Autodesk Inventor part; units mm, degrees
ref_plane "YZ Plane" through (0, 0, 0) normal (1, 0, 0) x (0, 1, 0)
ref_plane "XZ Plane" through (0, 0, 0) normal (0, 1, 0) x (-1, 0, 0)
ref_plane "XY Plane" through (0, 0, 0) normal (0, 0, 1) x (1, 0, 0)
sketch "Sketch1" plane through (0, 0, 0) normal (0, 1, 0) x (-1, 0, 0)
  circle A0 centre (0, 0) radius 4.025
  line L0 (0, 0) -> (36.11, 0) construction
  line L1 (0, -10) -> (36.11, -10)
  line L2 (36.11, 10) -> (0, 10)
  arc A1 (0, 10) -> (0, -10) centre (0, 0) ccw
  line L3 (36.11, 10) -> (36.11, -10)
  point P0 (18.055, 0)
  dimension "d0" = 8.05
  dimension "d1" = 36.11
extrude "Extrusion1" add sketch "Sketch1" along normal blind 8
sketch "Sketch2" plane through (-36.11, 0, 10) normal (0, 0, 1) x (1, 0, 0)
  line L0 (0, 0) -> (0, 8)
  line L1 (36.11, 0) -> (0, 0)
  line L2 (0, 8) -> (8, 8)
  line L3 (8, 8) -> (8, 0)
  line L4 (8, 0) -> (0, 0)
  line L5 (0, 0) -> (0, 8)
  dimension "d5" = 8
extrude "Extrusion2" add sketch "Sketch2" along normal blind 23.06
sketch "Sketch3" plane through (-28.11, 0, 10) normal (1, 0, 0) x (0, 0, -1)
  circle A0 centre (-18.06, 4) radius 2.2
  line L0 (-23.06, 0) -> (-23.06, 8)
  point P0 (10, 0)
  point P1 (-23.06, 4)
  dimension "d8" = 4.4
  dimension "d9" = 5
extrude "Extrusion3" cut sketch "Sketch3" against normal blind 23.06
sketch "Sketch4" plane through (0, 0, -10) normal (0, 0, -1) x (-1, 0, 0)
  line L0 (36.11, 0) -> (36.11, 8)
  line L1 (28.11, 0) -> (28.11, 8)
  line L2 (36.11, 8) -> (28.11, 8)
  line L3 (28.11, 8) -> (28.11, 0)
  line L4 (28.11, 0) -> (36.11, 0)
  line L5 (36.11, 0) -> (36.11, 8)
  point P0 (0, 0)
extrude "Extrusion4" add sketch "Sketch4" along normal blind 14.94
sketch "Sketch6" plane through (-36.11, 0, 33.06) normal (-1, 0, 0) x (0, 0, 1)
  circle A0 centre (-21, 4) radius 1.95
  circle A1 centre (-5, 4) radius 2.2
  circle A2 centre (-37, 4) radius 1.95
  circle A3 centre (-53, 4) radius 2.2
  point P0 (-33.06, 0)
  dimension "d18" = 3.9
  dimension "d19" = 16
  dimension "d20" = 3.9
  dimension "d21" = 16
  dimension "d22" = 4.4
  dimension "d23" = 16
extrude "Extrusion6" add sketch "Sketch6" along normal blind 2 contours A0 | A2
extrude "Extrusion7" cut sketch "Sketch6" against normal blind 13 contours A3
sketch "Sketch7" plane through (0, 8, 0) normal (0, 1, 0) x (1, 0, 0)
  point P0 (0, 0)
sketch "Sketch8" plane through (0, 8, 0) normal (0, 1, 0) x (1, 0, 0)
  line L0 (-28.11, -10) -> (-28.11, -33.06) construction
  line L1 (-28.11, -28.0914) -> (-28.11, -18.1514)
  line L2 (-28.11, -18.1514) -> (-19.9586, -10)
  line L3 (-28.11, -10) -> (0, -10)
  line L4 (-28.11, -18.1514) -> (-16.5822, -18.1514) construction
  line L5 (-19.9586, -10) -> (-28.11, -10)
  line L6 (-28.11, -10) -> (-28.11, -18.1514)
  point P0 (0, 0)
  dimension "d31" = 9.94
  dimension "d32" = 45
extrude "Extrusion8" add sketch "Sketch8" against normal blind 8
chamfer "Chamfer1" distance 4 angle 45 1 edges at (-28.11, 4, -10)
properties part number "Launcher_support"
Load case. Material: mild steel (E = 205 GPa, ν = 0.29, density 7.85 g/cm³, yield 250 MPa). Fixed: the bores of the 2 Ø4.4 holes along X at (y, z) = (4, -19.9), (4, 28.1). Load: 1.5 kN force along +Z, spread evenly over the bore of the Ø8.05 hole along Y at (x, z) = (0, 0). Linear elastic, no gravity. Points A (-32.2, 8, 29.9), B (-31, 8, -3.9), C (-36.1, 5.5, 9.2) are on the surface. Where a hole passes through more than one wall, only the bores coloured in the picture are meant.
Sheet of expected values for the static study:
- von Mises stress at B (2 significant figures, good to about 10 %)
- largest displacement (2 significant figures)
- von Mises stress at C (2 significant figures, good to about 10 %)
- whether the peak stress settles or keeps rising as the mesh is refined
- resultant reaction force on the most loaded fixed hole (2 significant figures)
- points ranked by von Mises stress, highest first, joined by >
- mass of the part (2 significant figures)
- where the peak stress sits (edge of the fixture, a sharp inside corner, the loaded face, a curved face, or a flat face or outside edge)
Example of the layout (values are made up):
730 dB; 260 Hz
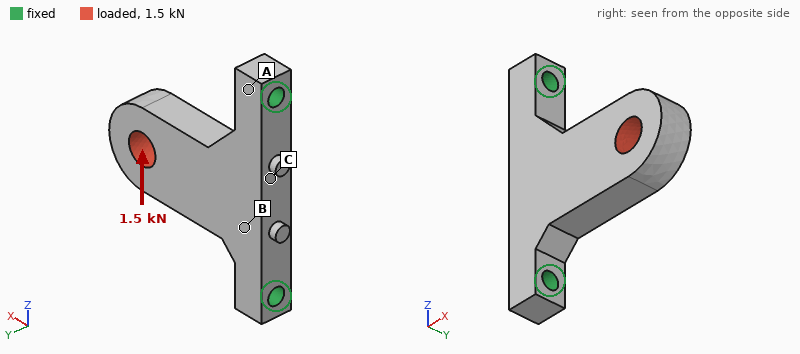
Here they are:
20 MPa; 31 µm; 40 MPa; keeps rising; 1.5 kN; C > B > A; 72 g; edge of the fixture
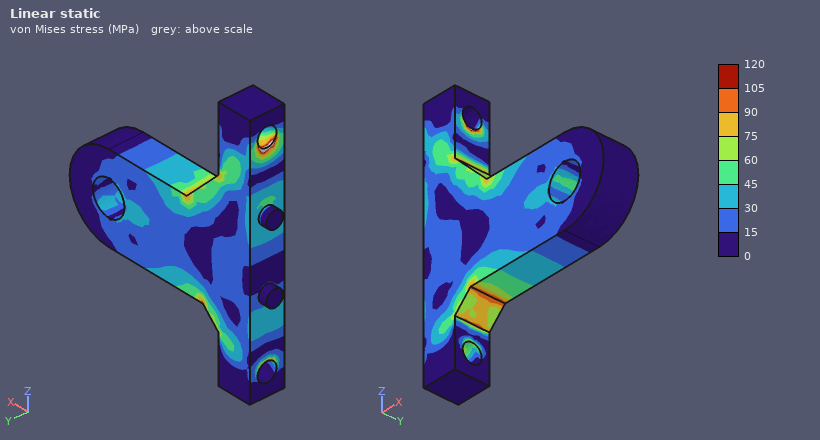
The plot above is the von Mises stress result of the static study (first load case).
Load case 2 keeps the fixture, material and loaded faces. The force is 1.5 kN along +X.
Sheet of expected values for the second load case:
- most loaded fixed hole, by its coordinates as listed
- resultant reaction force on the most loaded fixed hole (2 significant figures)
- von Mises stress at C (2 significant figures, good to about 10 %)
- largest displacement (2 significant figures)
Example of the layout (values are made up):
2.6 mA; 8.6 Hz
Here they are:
(4, -19.9); 980 N; 17 MPa; 5.6 µm
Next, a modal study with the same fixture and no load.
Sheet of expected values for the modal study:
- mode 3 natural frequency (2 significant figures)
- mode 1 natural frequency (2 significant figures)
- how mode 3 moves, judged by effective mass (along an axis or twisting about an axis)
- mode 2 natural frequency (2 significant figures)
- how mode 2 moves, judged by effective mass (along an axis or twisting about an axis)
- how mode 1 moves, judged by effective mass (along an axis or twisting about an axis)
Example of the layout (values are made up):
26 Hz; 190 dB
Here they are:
12 kHz; 2600 Hz; along Y; 8600 Hz; along Z; along Y
